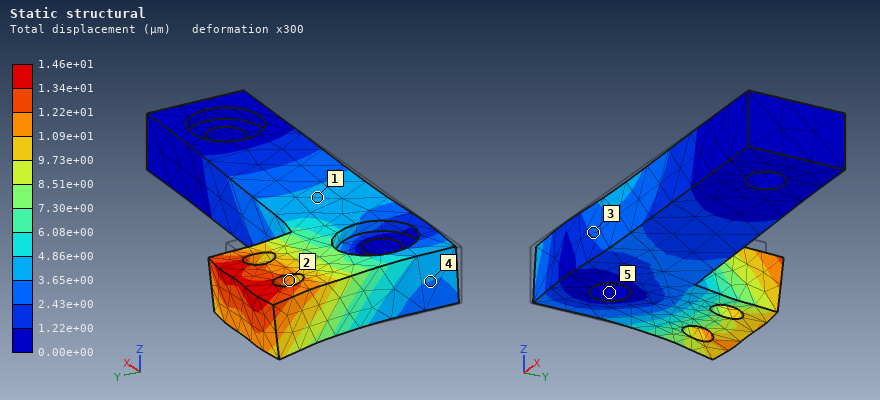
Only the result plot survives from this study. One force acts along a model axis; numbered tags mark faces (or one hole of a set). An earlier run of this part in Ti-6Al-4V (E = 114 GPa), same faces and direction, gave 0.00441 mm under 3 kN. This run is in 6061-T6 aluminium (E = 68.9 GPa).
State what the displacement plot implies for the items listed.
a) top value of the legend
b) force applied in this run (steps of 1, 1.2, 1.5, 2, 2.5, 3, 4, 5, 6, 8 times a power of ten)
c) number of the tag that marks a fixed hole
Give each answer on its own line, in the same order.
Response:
1.46e+01 µm
6 kN
5
